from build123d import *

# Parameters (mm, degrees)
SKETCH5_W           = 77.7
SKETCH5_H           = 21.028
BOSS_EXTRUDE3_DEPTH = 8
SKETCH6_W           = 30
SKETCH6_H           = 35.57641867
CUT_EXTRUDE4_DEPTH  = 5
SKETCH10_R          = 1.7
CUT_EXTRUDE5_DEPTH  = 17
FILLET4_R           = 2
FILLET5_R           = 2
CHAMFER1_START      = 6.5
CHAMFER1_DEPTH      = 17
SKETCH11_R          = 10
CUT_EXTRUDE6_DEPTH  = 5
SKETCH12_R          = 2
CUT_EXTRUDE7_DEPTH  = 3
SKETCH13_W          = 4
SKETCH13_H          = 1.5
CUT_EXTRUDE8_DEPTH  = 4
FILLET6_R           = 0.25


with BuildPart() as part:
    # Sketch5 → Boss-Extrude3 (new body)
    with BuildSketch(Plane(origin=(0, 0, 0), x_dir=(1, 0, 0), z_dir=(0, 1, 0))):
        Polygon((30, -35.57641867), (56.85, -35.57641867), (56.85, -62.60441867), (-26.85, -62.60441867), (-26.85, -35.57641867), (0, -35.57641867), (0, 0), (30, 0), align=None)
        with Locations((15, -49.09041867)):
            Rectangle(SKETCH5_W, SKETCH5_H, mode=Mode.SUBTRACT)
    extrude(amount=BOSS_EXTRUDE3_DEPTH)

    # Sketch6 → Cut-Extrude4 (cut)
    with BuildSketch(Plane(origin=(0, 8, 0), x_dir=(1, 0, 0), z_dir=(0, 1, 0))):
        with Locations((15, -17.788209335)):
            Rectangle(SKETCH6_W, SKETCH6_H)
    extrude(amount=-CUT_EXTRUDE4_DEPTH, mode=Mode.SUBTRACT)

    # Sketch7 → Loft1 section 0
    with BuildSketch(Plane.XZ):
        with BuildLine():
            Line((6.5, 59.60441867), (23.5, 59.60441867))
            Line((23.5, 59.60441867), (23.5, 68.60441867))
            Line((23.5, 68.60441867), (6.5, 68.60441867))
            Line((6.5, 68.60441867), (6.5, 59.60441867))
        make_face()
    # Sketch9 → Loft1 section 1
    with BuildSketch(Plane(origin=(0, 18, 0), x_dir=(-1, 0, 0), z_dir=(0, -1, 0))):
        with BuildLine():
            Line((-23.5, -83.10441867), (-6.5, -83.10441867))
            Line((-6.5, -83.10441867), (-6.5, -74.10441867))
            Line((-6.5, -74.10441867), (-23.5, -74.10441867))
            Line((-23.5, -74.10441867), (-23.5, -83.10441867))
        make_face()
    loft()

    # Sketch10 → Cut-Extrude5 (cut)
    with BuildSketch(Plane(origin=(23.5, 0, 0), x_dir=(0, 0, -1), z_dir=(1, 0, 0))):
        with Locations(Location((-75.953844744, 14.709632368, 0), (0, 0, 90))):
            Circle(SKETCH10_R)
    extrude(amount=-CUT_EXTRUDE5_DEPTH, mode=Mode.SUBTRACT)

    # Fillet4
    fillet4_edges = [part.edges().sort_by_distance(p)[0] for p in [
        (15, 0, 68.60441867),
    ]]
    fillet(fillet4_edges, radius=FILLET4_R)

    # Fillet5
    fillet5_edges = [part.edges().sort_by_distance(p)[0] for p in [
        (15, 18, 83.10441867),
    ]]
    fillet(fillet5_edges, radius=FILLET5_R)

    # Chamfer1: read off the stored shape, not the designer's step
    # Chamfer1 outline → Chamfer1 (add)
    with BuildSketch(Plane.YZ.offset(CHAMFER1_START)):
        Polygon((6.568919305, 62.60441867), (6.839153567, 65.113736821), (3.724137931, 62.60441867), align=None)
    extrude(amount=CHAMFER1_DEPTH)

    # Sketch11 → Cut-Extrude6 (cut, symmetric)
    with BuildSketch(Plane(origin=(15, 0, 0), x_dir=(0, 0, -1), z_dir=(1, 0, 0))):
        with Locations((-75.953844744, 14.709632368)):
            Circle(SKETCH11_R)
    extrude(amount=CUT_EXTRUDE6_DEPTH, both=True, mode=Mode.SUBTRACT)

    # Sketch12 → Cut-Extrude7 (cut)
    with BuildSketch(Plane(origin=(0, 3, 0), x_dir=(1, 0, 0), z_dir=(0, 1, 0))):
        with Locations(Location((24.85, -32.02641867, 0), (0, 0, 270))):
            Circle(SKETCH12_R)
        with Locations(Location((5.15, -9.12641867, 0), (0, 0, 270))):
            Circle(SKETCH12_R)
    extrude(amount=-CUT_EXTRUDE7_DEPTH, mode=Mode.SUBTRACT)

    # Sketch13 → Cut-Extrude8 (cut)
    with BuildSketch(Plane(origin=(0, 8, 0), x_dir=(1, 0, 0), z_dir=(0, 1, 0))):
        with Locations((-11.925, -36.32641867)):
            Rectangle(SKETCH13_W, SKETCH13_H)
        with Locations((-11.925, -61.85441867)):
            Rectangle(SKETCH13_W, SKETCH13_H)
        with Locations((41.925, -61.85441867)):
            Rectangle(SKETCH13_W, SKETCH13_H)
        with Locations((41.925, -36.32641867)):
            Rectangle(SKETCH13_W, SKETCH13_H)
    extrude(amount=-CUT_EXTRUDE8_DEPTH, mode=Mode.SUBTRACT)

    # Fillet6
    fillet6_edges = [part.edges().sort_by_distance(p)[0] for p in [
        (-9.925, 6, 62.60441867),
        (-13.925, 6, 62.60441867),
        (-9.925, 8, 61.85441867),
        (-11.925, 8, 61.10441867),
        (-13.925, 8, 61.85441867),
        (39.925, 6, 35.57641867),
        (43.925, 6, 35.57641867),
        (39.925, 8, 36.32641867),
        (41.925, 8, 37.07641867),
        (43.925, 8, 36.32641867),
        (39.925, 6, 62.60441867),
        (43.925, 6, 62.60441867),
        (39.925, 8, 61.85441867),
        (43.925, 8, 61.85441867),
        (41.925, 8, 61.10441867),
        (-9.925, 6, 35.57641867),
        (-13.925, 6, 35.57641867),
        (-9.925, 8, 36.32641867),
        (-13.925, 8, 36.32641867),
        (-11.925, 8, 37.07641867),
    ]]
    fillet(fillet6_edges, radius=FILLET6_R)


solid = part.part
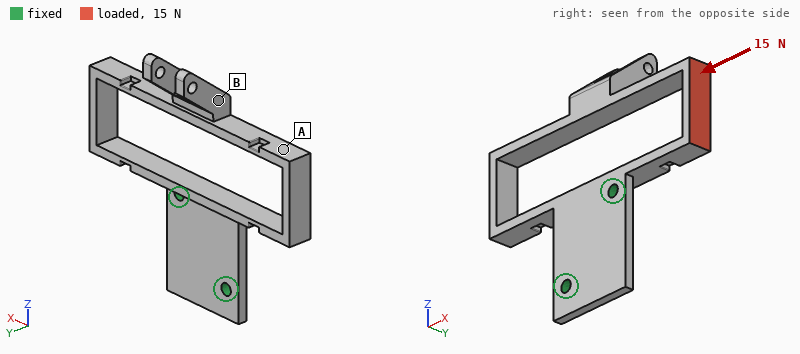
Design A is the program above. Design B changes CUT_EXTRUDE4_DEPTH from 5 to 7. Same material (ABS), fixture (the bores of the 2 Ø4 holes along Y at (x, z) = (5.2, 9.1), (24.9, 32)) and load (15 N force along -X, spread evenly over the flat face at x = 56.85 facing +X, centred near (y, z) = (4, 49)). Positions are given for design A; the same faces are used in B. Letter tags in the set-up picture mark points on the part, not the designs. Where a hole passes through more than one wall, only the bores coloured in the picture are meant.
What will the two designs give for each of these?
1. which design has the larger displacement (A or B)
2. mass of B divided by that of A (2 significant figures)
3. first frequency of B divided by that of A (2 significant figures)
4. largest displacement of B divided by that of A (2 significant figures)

B
0.79
0.57
1.2
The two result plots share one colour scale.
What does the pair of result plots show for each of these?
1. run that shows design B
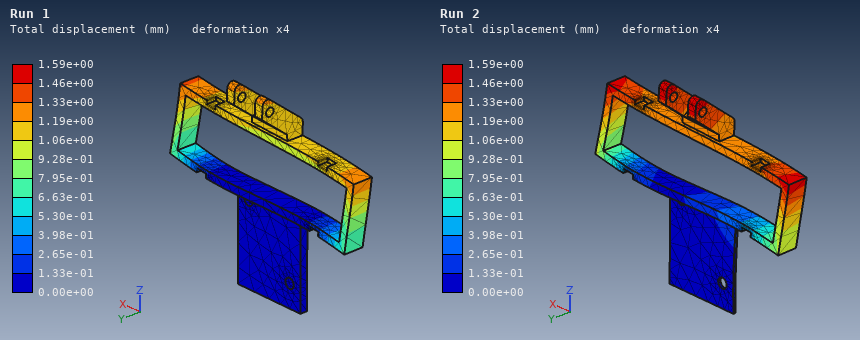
Run 2
